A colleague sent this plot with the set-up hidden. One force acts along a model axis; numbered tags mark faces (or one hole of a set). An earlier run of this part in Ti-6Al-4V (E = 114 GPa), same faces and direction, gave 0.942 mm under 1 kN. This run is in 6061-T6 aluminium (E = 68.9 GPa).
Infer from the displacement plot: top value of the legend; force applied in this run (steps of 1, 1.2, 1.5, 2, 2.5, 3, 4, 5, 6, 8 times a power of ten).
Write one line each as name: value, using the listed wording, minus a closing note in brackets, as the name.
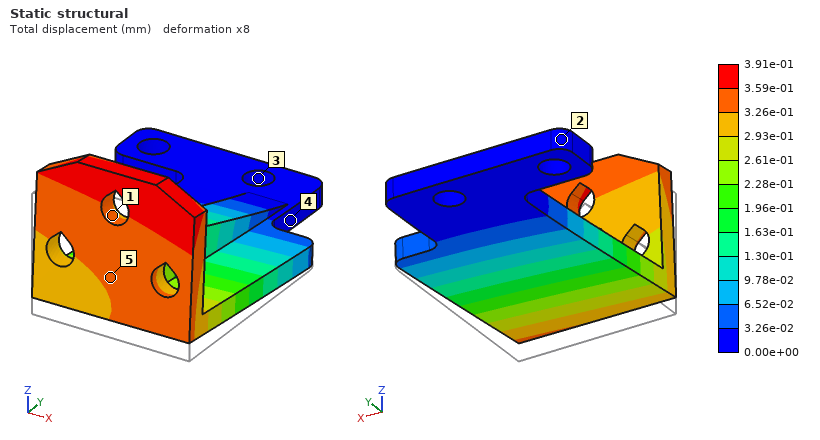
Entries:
top value of the legend: 3.91e-01 mm
force applied in this run: 250 N
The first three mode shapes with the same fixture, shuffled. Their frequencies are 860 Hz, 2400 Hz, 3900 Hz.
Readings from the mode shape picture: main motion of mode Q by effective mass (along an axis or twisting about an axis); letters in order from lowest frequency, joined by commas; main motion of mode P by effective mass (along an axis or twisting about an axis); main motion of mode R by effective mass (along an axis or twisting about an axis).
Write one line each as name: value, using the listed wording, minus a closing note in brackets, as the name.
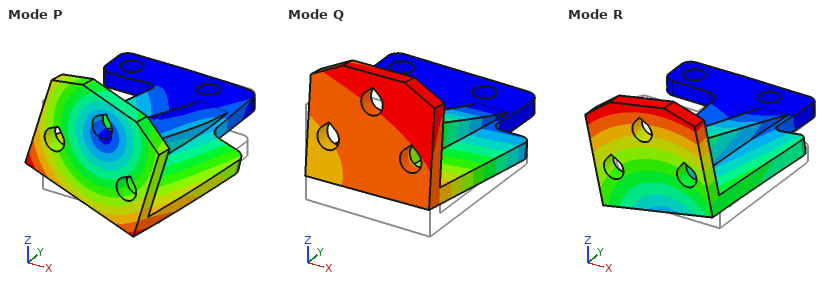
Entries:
main motion of mode Q by effective mass: along Z
letters in order from lowest frequency, joined by commas: Q, R, P
main motion of mode P by effective mass: along X
main motion of mode R by effective mass: along X
